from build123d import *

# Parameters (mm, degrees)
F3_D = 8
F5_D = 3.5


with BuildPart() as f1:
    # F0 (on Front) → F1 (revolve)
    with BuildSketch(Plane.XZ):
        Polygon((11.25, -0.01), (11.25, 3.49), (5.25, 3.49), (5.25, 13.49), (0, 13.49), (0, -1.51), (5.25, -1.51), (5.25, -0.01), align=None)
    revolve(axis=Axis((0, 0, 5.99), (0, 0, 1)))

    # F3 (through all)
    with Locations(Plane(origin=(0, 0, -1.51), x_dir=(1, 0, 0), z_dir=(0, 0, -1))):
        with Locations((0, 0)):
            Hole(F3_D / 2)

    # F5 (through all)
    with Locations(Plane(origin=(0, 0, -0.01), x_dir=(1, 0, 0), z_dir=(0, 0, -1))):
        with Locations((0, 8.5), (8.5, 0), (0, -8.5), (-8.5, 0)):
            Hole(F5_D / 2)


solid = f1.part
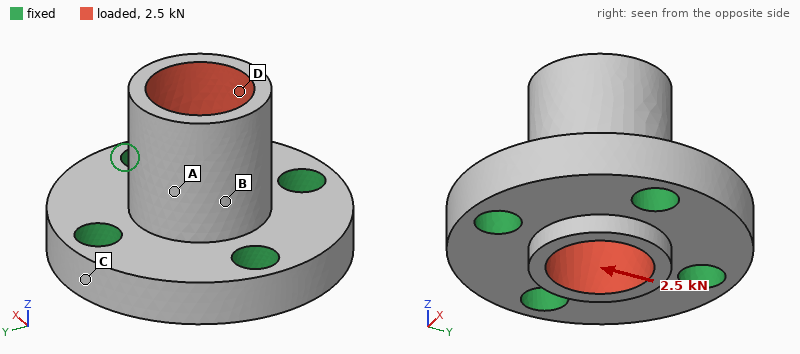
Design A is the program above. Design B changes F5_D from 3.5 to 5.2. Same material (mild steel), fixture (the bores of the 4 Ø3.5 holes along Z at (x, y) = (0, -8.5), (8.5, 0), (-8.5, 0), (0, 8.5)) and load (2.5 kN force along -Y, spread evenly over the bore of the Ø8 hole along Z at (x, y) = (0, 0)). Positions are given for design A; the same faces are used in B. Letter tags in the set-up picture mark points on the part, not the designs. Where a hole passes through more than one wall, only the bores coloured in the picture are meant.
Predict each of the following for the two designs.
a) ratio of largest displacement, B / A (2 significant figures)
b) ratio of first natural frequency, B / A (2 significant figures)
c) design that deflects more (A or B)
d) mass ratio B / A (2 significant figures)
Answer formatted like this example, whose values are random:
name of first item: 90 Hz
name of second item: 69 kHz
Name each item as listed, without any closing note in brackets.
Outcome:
ratio of largest displacement, B / A: 0.89
ratio of first natural frequency, B / A: 1.1
design that deflects more: A
mass ratio B / A: 0.89
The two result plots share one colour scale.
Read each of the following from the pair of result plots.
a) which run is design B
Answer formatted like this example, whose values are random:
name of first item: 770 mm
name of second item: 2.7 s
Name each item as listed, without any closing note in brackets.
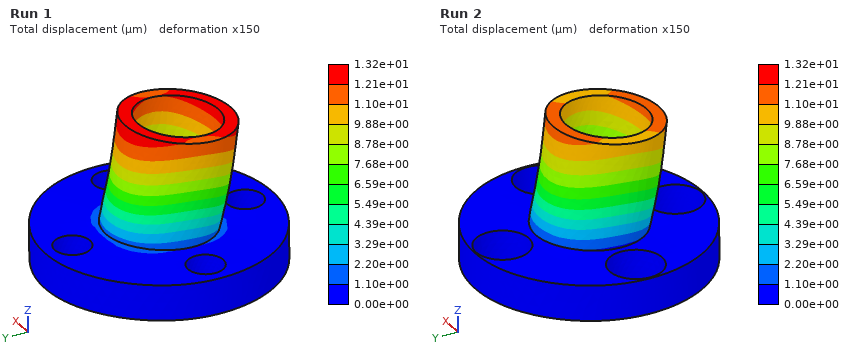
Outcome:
which run is design B: Run 2
